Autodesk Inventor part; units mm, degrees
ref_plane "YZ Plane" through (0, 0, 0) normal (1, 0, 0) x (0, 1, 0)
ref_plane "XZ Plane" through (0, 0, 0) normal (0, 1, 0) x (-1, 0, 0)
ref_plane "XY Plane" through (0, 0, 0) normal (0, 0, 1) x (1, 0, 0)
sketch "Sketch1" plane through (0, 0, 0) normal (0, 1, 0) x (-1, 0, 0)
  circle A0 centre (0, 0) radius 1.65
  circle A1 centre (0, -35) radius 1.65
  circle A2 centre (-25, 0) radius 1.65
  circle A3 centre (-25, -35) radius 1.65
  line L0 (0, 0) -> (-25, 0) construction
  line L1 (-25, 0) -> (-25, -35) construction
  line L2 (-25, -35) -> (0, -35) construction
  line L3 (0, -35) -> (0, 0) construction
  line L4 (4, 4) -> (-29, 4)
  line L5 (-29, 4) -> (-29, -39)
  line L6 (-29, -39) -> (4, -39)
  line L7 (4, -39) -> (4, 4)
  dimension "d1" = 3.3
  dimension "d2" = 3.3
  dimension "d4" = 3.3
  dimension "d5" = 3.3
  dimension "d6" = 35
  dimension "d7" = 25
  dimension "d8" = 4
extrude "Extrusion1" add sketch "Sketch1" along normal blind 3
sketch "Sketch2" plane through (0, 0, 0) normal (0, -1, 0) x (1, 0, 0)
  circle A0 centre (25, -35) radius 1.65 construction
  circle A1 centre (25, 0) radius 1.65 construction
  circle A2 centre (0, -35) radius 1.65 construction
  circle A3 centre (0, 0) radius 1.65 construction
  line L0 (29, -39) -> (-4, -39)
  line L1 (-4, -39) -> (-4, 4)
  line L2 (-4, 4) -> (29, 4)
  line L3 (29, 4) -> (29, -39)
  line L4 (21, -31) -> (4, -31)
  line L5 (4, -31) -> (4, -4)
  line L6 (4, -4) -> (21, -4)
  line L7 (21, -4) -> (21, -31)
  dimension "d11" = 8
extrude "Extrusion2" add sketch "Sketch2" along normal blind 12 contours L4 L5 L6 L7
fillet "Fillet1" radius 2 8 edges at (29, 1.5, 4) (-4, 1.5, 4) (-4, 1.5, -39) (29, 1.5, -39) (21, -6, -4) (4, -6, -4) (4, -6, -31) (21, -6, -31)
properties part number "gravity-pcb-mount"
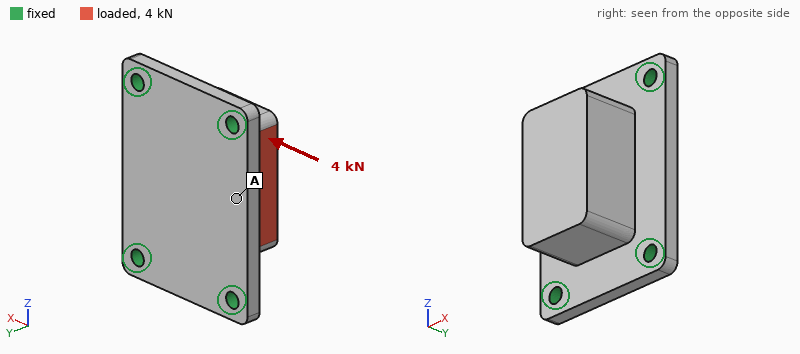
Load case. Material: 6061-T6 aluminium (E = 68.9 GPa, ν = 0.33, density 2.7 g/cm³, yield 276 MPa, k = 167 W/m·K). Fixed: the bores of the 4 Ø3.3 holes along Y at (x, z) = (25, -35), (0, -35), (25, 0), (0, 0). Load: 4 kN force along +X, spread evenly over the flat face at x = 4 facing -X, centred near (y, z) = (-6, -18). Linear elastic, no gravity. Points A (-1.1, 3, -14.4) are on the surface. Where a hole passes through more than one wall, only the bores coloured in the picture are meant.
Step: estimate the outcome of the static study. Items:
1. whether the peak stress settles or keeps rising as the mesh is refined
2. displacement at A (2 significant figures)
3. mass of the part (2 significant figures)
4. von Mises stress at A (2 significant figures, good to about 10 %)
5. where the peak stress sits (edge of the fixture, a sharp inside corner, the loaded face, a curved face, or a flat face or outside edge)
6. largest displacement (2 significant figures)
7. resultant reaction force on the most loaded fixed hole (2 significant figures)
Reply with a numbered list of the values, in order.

1. keeps rising
2. 33 µm
3. 26 g
4. 41 MPa
5. edge of the fixture
6. 54 µm
7. 1.3 kN
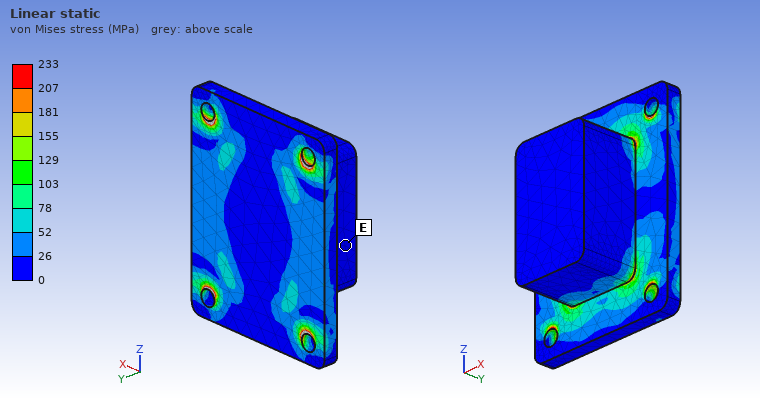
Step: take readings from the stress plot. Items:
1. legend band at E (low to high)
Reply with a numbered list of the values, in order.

1. 0 to 26 MPa
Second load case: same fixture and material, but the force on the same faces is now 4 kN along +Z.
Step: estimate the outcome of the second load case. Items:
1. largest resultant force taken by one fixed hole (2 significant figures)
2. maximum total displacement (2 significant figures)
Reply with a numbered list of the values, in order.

1. 1.3 kN
2. 34 µm
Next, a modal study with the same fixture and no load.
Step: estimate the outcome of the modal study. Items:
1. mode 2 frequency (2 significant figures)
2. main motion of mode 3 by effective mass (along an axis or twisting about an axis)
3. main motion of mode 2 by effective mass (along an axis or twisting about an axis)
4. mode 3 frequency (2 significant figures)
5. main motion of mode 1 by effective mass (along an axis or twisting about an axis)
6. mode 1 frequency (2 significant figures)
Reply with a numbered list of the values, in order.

1. 12 kHz
2. along Z
3. along X
4. 15 kHz
5. along Y
6. 11 kHz
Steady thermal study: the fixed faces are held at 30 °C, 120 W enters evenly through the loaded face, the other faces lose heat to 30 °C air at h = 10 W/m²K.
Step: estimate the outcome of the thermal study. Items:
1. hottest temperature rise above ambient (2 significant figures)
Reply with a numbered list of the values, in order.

1. 68 K
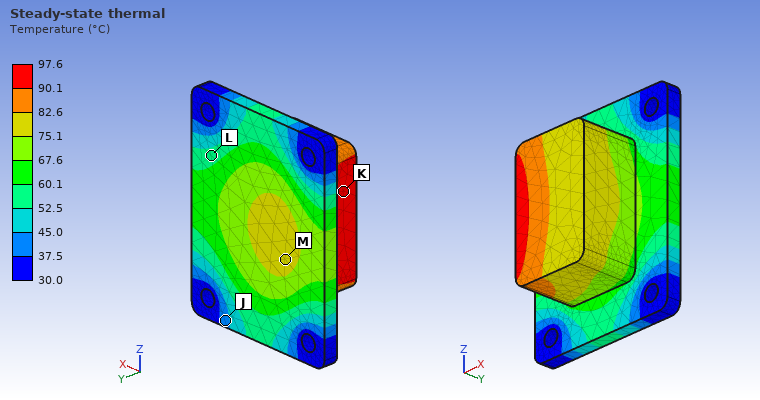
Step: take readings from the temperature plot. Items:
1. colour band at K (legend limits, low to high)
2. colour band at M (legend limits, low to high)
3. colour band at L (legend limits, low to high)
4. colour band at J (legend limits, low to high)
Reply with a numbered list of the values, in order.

1. 90.1 to 97.6 °C
2. 75.1 to 82.6 °C
3. 52.5 to 60.1 °C
4. 37.5 to 45.0 °C
